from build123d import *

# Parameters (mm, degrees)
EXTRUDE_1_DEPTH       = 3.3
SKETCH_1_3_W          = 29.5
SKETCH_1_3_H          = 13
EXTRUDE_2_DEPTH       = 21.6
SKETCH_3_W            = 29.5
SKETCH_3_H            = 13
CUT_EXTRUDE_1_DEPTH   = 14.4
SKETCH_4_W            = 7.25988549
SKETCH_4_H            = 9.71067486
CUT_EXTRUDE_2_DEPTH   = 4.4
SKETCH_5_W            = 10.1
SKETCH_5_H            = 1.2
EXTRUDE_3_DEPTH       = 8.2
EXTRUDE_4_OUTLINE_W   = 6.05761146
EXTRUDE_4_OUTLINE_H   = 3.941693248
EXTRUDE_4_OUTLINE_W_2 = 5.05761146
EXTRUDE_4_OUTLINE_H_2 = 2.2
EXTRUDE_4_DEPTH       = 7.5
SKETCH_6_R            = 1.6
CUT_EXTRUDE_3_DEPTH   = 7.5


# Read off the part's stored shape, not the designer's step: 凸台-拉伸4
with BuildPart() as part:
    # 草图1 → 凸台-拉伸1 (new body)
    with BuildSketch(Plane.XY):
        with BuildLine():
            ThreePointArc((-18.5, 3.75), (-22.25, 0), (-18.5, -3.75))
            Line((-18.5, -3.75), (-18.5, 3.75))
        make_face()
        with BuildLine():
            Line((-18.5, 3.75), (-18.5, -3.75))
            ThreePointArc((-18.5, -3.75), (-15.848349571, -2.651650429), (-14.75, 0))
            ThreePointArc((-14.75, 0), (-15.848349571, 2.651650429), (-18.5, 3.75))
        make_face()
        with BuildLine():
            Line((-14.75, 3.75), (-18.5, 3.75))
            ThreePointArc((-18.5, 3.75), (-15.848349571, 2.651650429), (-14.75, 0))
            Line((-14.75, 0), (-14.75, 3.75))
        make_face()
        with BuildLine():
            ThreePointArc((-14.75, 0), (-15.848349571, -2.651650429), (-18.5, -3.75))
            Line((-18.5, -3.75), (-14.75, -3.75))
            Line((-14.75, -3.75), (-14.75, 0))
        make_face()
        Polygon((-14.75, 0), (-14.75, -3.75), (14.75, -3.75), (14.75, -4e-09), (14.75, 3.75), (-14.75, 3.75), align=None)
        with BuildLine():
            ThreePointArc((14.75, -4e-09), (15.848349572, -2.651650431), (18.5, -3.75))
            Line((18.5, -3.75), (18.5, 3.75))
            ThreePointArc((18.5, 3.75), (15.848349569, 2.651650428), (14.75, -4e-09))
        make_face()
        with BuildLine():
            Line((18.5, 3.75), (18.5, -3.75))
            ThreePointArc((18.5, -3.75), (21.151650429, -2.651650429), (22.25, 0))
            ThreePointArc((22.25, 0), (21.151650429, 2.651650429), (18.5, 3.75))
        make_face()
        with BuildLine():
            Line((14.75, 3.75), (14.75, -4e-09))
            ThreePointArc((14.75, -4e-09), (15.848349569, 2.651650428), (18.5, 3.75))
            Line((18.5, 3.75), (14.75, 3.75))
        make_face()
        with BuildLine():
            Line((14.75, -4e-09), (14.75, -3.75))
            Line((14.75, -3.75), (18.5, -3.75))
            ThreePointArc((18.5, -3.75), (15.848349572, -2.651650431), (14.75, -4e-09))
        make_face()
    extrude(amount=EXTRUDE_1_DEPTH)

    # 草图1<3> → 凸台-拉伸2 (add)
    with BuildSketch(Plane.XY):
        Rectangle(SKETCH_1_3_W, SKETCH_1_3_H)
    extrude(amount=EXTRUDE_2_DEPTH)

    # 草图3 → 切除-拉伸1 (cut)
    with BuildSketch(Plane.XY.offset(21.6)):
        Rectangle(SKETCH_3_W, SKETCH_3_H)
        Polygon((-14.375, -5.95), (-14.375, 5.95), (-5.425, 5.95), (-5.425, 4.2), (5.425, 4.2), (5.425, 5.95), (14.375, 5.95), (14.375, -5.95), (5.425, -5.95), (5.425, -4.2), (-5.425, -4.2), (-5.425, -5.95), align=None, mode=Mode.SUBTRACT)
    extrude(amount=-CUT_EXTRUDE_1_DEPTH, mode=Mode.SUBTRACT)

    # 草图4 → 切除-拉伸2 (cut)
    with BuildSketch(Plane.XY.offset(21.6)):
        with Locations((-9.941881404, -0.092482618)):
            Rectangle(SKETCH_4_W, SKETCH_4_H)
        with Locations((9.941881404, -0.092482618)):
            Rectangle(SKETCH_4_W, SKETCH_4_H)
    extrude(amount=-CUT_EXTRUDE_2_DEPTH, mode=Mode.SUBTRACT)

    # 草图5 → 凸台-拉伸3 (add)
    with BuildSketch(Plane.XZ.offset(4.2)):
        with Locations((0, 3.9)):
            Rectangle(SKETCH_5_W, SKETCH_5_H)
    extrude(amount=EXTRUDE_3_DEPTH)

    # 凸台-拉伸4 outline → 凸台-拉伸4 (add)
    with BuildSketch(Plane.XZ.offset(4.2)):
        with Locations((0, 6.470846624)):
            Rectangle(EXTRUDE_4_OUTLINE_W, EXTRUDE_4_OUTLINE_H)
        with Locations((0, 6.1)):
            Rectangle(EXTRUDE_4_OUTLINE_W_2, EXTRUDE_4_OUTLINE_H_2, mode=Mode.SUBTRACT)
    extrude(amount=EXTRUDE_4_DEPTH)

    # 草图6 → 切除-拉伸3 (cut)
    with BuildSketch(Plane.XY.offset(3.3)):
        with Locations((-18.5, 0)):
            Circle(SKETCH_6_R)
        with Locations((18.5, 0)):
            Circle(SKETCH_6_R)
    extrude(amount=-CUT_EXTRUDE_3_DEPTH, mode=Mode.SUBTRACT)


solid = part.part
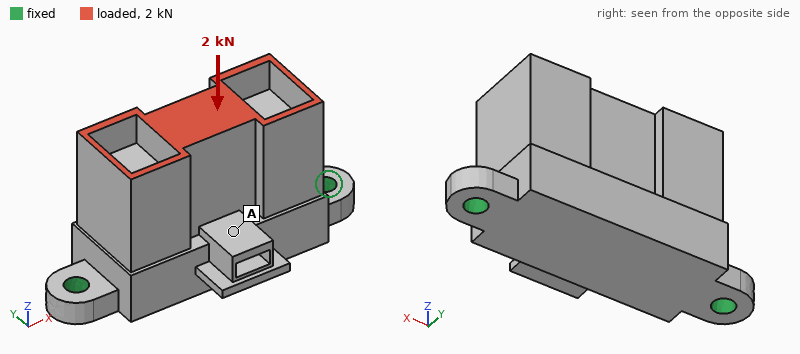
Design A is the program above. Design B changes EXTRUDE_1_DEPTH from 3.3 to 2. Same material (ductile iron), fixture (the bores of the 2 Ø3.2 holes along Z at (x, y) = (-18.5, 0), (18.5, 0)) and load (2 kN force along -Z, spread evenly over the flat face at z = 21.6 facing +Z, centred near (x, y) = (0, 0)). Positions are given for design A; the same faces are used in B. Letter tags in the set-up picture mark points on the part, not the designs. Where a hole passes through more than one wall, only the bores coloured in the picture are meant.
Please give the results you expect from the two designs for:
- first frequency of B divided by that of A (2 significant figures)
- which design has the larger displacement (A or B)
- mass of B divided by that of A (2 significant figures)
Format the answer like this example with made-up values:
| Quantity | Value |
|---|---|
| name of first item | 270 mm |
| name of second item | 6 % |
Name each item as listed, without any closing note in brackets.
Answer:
| Quantity | Value |
|---|---|
| first frequency of B divided by that of A | 0.59 |
| which design has the larger displacement | B |
| mass of B divided by that of A | 0.98 |
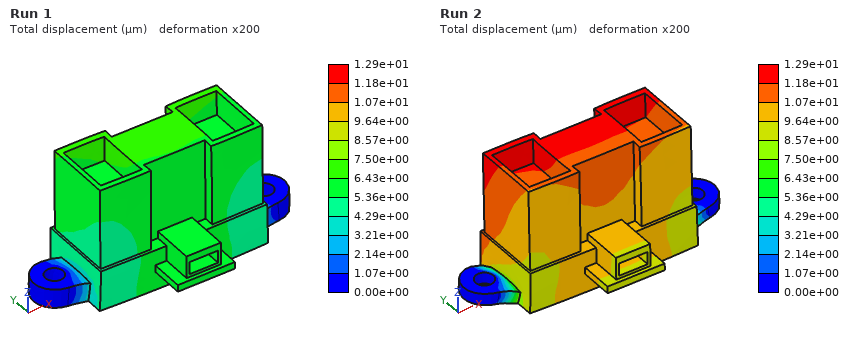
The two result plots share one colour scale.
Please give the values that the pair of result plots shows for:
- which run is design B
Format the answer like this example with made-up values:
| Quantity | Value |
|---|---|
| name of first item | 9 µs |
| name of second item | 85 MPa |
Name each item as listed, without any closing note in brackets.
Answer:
| Quantity | Value |
|---|---|
| which run is design B | Run 2 |
